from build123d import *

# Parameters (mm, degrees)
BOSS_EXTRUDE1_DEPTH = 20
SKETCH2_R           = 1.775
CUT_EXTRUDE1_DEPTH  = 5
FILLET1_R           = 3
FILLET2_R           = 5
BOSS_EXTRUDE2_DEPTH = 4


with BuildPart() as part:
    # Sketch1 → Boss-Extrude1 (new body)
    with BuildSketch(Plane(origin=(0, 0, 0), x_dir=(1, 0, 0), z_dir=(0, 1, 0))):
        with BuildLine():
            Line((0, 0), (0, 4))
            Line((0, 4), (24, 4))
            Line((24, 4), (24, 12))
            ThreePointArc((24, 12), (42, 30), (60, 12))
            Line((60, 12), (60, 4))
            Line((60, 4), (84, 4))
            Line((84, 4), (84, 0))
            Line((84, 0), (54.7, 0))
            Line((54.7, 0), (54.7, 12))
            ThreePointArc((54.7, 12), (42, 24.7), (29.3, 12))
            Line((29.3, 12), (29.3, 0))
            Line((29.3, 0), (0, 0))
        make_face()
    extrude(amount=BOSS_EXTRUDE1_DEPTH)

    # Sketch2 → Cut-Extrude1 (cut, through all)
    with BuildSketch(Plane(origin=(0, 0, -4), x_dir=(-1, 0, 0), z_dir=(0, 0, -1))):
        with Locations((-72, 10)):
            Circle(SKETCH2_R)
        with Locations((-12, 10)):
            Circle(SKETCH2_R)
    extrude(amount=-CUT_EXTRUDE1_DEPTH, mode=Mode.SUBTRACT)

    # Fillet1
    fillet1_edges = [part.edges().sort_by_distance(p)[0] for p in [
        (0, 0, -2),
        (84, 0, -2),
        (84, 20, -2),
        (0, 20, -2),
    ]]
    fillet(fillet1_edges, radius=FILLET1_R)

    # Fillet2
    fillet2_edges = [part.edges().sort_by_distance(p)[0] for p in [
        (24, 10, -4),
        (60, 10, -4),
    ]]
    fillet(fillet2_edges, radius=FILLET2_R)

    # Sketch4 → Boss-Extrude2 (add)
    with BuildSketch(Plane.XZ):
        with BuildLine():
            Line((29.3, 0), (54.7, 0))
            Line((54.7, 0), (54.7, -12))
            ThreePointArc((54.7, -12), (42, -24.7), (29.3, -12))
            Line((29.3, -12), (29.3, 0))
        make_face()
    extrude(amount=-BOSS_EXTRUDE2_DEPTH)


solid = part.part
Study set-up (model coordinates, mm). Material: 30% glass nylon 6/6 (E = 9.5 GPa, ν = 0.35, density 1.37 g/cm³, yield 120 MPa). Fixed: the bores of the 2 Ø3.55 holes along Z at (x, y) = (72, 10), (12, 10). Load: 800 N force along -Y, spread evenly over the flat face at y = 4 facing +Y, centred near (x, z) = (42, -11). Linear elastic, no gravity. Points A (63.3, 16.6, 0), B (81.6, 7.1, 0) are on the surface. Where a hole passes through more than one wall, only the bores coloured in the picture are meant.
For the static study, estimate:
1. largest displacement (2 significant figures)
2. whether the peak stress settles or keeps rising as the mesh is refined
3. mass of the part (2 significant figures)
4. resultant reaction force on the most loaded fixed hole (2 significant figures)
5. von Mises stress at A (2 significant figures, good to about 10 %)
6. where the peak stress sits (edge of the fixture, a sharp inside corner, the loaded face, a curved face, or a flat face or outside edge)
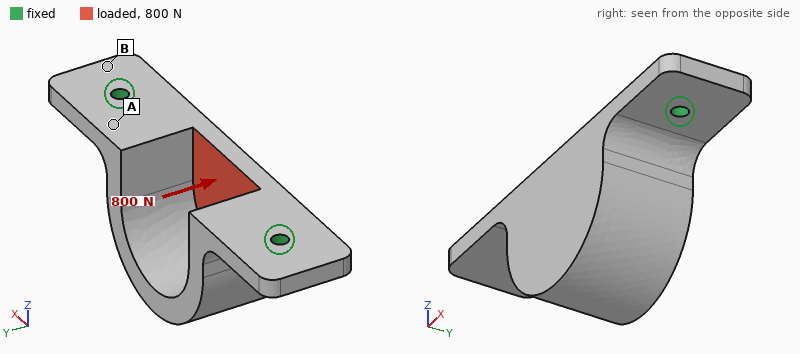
0.84 mm
keeps rising
19 g
610 N
24 MPa
edge of the fixture
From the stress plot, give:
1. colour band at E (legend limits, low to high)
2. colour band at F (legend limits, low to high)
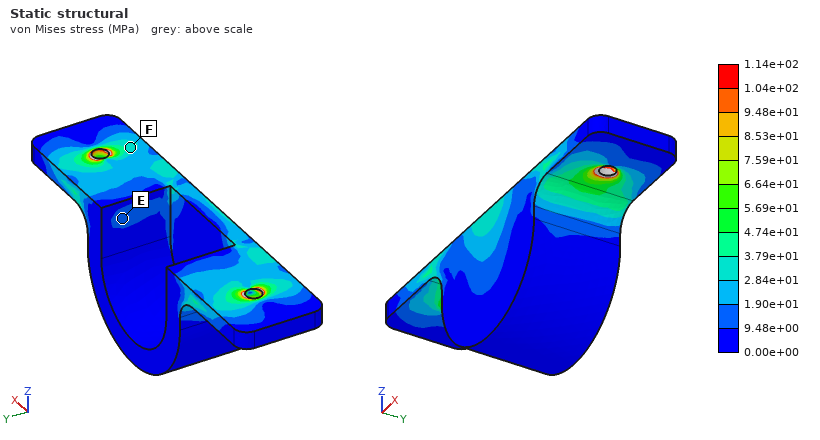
9.48e+00 to 1.90e+01 MPa
2.84e+01 to 3.79e+01 MPa
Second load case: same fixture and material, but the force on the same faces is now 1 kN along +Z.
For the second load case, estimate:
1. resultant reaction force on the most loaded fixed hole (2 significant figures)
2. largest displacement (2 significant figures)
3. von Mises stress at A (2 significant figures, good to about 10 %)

570 N
0.66 mm
22 MPa
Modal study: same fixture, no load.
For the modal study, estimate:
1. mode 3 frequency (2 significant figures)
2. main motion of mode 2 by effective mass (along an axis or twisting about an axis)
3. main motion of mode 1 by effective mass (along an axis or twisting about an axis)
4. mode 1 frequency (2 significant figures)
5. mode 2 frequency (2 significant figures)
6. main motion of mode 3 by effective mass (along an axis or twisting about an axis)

4500 Hz
along Z
along Y
1300 Hz
3600 Hz
along X
